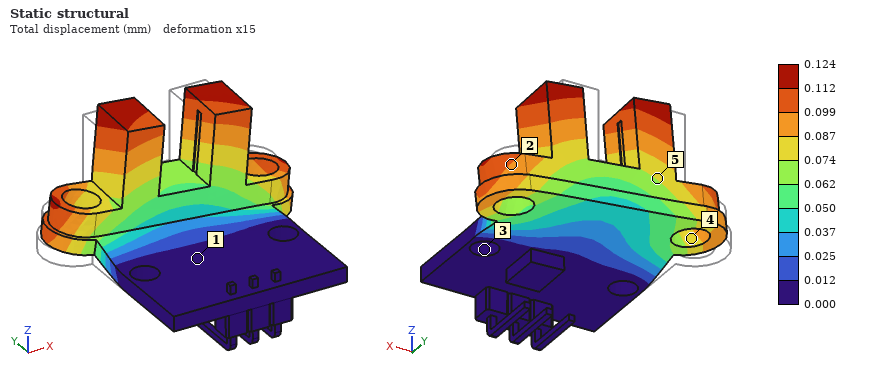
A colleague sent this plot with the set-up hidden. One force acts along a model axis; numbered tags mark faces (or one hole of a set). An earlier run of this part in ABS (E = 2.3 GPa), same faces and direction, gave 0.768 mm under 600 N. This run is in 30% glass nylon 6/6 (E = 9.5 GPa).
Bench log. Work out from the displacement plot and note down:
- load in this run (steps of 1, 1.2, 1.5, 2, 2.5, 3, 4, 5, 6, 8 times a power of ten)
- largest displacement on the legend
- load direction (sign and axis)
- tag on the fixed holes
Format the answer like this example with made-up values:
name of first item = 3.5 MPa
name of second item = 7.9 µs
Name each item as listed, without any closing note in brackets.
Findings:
load in this run = 400 N
largest displacement on the legend = 0.124 mm
load direction = +X
tag on the fixed holes = 3
